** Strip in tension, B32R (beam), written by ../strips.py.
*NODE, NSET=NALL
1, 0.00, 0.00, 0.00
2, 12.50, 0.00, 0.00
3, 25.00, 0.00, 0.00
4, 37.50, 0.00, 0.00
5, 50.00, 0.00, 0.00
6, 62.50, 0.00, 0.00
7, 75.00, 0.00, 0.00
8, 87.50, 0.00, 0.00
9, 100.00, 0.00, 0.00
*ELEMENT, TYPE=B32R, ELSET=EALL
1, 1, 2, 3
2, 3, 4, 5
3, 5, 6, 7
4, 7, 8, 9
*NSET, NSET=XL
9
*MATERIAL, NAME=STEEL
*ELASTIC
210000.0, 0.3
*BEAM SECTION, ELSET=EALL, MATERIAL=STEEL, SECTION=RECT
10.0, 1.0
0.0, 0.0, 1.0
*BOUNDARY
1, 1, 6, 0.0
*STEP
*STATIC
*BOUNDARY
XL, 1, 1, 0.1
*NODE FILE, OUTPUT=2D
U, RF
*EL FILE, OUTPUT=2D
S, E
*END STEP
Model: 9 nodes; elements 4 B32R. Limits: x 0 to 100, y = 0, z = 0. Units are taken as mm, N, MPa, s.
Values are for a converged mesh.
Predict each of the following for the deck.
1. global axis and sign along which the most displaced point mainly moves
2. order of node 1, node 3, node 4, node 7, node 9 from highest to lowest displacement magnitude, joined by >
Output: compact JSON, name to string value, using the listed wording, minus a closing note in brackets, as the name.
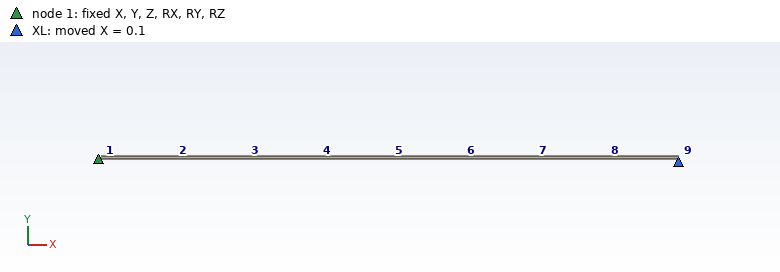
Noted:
{"global axis and sign along which the most displaced point mainly moves": "+X", "order of node 1, node 3, node 4, node 7, node 9 from highest to lowest displacement magnitude, joined by >": "node 9 > node 7 > node 4 > node 3 > node 1"}
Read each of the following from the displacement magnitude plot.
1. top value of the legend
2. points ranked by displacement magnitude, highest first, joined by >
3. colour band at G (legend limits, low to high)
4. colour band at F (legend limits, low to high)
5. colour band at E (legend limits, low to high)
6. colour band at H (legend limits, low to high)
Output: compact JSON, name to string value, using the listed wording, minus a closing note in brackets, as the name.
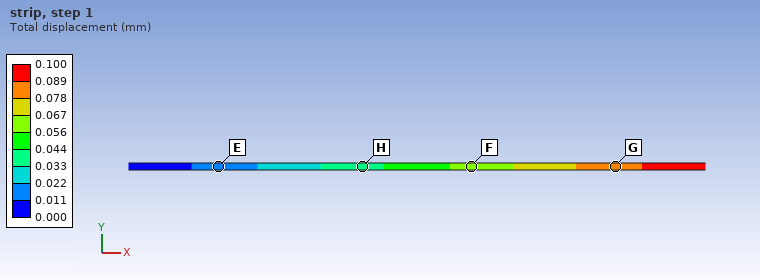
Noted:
{"top value of the legend": "0.100 mm", "points ranked by displacement magnitude, highest first, joined by >": "G > F > H > E", "colour band at G": "0.078 to 0.089 mm", "colour band at F": "0.056 to 0.067 mm", "colour band at E": "0.011 to 0.022 mm", "colour band at H": "0.033 to 0.044 mm"}
